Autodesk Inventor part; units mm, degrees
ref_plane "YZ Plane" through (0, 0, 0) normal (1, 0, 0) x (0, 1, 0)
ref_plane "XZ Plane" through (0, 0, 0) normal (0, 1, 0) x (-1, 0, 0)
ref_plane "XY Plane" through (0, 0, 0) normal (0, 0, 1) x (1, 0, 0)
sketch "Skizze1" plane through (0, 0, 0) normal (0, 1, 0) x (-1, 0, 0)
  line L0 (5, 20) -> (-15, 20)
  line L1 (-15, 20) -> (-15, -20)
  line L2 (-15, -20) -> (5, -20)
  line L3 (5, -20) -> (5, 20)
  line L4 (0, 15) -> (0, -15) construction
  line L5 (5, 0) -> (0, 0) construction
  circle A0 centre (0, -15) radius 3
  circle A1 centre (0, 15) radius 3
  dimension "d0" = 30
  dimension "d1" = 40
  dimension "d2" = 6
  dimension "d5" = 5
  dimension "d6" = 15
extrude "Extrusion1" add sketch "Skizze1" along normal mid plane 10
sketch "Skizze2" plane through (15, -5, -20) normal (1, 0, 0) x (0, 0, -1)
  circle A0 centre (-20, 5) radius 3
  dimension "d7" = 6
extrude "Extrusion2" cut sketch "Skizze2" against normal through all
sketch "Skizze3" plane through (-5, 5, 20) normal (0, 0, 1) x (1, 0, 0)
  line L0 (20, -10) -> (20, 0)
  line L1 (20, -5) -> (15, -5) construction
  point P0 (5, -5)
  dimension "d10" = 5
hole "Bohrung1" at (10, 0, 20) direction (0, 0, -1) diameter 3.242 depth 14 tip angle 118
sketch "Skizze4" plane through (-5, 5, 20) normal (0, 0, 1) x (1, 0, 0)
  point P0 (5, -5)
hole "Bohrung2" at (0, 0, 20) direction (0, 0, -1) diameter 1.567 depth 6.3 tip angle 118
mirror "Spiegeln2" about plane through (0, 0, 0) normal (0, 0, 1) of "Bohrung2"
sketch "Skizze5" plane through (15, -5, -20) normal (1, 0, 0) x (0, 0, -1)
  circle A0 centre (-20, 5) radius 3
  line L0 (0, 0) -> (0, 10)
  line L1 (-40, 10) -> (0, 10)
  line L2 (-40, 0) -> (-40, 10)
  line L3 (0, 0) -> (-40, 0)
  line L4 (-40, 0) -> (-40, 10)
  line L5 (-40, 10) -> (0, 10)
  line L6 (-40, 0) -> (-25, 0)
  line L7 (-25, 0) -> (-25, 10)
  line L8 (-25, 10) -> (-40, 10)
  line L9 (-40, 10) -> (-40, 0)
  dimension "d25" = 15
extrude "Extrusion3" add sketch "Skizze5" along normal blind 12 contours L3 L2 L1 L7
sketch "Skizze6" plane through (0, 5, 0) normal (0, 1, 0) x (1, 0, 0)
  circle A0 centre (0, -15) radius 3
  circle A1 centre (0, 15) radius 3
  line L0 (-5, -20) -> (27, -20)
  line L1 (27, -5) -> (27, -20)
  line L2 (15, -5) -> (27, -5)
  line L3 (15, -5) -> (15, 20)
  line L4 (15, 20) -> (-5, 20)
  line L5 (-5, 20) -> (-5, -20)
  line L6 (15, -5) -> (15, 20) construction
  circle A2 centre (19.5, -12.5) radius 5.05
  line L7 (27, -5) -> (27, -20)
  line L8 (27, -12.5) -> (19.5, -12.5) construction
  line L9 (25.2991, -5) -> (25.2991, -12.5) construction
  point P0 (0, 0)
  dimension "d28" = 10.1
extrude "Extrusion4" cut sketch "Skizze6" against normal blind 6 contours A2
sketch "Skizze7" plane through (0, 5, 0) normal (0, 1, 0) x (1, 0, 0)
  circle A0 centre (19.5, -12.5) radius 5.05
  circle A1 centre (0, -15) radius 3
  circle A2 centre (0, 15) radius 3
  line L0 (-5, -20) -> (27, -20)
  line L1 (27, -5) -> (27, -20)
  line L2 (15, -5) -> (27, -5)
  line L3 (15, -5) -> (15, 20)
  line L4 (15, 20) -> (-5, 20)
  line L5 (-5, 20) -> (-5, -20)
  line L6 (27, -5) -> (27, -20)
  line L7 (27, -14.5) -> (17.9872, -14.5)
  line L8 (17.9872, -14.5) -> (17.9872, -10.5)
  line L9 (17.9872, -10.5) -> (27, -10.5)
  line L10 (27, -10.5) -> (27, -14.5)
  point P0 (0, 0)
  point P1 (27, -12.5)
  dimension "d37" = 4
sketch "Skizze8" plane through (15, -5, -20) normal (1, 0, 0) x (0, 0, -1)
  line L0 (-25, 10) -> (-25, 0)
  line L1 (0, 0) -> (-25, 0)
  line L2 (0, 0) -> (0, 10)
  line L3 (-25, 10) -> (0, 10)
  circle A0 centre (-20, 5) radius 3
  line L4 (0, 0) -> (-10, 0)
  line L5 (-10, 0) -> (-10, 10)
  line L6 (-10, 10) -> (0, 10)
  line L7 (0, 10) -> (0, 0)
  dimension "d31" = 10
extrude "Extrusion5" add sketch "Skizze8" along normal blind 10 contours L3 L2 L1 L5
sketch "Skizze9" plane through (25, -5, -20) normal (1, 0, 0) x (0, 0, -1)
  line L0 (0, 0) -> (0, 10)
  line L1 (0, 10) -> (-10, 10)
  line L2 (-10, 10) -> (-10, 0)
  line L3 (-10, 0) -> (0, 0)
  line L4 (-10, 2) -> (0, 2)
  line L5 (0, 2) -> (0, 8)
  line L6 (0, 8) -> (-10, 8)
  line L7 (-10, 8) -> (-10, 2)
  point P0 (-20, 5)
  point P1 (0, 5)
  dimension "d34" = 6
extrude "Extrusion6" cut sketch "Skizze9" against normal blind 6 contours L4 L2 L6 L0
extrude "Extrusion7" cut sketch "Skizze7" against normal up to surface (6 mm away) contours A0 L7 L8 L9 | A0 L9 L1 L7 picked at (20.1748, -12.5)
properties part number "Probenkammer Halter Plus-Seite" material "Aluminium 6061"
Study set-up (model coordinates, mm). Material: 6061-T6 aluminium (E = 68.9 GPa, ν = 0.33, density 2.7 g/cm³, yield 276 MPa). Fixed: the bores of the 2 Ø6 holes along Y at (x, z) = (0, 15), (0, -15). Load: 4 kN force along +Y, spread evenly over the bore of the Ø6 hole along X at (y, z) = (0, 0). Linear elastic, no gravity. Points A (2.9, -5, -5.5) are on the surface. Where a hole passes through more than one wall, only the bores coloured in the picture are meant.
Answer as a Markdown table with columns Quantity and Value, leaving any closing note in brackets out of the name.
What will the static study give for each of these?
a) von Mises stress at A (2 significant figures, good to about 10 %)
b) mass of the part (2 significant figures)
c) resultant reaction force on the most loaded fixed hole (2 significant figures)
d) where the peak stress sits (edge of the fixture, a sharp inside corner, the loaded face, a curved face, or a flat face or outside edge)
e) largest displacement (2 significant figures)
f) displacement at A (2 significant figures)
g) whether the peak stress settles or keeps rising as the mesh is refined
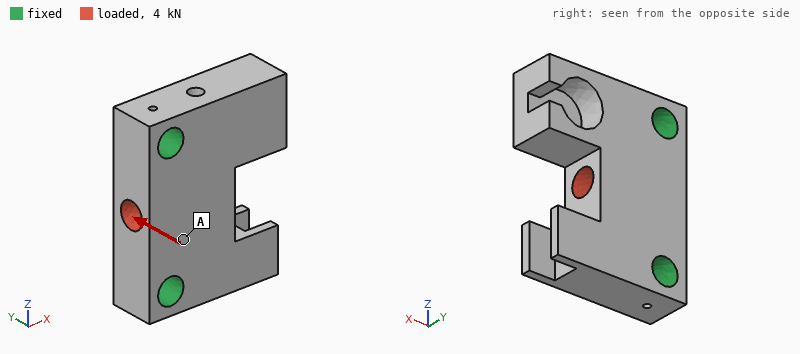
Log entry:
| Quantity | Value |
|---|---|
| von Mises stress at A | 14 MPa |
| mass of the part | 23 g |
| resultant reaction force on the most loaded fixed hole | 2.0 kN |
| where the peak stress sits | edge of the fixture |
| largest displacement | 25 µm |
| displacement at A | 8.8 µm |
| whether the peak stress settles or keeps rising as the mesh is refined | keeps rising |
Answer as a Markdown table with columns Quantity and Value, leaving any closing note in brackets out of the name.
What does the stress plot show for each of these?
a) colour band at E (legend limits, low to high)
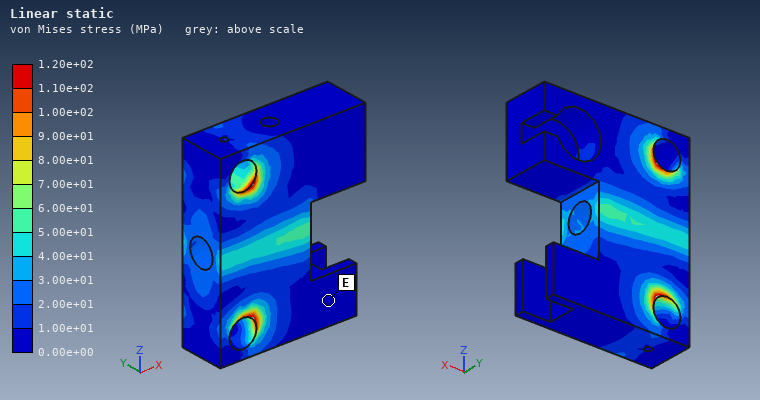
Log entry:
| Quantity | Value |
|---|---|
| colour band at E | 0.00e+00 to 1.00e+01 MPa |
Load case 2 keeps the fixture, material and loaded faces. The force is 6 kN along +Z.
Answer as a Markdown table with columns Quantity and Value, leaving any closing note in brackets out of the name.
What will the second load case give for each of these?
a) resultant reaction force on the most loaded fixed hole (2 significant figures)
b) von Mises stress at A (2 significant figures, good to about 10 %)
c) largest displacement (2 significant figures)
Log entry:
| Quantity | Value |
|---|---|
| resultant reaction force on the most loaded fixed hole | 3.1 kN |
| von Mises stress at A | 21 MPa |
| largest displacement | 7.8 µm |
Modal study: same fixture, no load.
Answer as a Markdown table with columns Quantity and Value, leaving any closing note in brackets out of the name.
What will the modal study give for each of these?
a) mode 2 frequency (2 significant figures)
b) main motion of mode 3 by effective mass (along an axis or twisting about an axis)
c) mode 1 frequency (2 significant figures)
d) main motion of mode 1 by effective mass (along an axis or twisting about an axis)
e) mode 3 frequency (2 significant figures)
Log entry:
| Quantity | Value |
|---|---|
| mode 2 frequency | 18 kHz |
| main motion of mode 3 by effective mass | along Z |
| mode 1 frequency | 13 kHz |
| main motion of mode 1 by effective mass | along Y |
| mode 3 frequency | 19 kHz |
